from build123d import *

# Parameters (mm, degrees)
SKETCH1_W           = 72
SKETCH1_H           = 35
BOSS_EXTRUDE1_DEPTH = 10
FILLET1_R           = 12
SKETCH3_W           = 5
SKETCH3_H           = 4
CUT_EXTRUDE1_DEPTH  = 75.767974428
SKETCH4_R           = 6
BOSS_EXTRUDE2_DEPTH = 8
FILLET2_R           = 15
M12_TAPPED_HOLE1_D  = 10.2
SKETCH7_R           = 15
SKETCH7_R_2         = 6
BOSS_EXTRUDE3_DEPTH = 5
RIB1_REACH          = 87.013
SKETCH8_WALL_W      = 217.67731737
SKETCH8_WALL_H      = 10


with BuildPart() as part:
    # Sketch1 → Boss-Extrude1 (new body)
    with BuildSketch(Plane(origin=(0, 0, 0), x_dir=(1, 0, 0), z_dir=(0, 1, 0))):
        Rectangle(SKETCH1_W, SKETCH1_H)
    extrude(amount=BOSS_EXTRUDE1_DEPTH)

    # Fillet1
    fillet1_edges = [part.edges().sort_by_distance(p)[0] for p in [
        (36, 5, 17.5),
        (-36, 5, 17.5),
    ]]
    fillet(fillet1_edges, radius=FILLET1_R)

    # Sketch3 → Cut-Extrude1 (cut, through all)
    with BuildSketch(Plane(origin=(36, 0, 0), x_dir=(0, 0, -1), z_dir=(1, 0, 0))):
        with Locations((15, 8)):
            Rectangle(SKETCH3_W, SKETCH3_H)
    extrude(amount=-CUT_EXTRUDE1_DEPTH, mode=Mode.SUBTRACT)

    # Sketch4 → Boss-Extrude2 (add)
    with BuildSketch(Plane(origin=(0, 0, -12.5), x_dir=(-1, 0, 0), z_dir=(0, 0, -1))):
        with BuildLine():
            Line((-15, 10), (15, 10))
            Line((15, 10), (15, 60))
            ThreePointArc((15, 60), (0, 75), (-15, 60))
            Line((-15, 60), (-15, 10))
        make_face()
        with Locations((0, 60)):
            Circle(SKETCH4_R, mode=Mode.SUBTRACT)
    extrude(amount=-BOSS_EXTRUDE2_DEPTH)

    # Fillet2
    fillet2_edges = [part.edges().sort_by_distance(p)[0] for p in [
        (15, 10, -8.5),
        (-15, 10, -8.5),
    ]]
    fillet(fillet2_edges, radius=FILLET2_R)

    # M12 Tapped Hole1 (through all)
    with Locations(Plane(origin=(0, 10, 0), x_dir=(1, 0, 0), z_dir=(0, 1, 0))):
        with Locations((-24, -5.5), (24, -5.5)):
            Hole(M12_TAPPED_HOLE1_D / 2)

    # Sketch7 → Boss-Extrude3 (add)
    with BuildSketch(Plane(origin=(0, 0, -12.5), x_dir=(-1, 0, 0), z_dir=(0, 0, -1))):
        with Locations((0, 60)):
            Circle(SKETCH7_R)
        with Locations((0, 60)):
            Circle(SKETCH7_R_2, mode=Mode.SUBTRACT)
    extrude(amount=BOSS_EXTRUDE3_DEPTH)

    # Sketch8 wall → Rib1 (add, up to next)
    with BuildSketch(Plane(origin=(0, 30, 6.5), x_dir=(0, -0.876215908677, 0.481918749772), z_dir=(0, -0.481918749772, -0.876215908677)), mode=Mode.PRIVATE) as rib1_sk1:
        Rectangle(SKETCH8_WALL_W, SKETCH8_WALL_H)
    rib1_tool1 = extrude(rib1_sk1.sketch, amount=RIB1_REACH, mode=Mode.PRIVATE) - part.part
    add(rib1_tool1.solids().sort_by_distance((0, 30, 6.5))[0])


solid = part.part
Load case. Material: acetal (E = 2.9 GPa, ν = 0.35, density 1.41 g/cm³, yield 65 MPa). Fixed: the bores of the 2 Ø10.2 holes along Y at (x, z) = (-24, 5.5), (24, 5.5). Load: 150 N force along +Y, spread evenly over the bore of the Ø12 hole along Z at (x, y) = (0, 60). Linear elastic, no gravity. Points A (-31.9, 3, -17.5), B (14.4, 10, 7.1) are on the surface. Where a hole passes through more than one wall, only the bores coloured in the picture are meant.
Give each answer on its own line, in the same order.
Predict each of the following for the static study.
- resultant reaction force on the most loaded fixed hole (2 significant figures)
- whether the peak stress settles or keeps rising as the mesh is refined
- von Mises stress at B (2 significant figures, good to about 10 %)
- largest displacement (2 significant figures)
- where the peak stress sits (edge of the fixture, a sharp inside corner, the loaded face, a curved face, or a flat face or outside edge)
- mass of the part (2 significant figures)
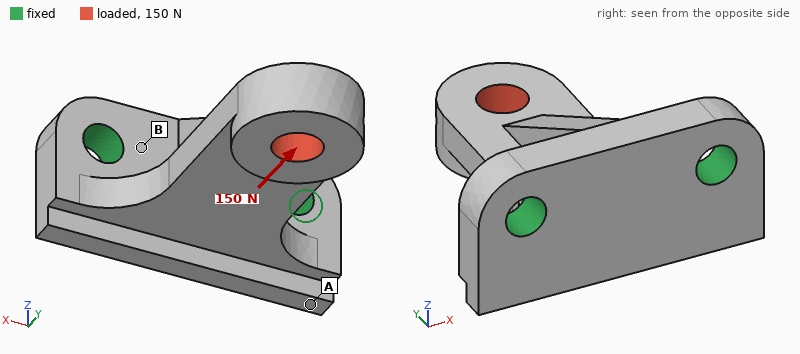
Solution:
77 N
keeps rising
0.98 MPa
0.15 mm
edge of the fixture
61 g
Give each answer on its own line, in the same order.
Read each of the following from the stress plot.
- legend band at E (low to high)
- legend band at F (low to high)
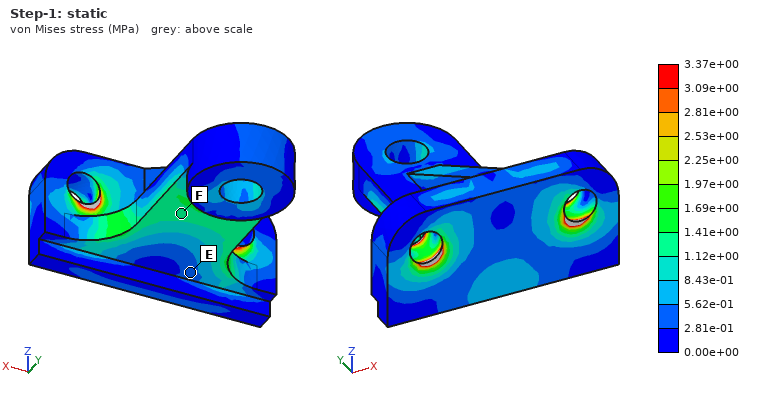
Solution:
2.81e-01 to 5.62e-01 MPa
1.12e+00 to 1.41e+00 MPa
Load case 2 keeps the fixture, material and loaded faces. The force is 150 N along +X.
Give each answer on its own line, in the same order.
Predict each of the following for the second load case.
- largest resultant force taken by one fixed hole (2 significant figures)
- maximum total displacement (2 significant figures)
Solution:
210 N
0.25 mm
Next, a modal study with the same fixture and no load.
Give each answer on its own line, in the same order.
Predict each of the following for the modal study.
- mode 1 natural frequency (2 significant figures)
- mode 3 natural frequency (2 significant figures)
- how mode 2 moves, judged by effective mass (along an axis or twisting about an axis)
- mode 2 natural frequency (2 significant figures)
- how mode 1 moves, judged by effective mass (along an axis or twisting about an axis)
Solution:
710 Hz
2200 Hz
along X
1200 Hz
along Z
